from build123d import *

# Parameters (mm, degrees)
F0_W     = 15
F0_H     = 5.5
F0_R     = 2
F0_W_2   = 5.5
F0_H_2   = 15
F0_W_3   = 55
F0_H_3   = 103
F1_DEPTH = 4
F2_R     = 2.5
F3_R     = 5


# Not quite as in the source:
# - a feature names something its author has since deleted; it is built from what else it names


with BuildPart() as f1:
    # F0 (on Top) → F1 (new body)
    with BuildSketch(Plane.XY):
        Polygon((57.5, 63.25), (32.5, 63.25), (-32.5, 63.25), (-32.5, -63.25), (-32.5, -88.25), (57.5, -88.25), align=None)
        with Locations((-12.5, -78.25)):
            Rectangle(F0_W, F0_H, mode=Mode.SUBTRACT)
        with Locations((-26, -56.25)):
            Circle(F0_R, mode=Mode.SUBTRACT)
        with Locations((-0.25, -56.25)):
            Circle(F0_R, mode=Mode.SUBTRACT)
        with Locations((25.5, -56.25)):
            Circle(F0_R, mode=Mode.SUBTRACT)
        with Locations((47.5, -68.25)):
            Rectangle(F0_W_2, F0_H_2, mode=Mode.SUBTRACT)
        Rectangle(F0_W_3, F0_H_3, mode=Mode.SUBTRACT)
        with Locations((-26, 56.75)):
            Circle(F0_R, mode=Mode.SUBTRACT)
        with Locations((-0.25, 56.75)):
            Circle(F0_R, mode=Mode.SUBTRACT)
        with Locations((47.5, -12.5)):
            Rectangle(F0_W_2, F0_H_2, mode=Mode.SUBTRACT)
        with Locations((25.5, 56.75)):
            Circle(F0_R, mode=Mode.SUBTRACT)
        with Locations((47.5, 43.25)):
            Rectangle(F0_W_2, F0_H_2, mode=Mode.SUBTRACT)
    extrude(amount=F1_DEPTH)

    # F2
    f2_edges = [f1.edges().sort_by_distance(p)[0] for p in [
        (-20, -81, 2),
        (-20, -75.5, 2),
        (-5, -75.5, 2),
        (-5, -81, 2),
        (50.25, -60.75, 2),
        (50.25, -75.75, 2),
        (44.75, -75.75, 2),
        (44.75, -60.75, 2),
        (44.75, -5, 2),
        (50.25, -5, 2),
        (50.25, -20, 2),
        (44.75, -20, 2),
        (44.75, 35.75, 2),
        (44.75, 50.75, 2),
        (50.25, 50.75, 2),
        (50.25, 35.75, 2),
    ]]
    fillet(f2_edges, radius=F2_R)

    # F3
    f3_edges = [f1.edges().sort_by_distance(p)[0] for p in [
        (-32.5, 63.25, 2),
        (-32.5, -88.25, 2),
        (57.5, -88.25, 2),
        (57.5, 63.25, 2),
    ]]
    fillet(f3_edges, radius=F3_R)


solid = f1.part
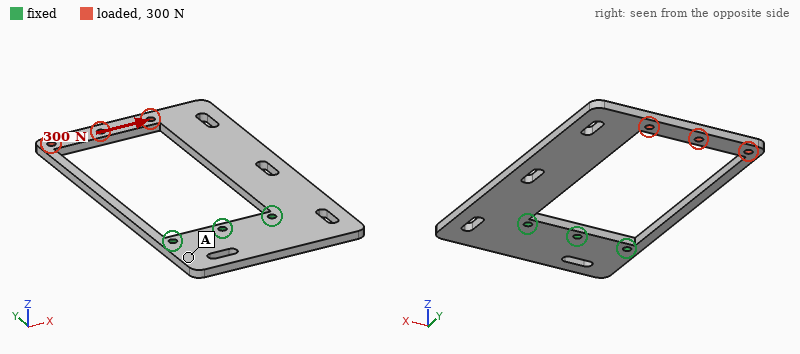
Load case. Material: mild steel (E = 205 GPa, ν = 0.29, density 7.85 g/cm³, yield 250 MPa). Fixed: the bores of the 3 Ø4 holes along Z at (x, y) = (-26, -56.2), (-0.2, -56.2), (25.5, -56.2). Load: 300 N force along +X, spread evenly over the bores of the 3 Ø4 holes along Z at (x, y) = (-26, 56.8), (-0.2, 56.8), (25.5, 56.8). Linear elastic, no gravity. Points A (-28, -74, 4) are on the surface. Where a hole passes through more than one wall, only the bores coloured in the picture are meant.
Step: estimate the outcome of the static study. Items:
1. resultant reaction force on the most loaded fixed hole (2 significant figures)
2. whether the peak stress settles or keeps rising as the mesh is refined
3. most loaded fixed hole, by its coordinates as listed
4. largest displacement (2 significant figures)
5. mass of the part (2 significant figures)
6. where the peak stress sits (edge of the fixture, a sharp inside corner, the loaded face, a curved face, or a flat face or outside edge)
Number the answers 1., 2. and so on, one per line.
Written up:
1. 1.2 kN
2. keeps rising
3. (25.5, -56.2)
4. 0.12 mm
5. 240 g
6. a sharp inside corner
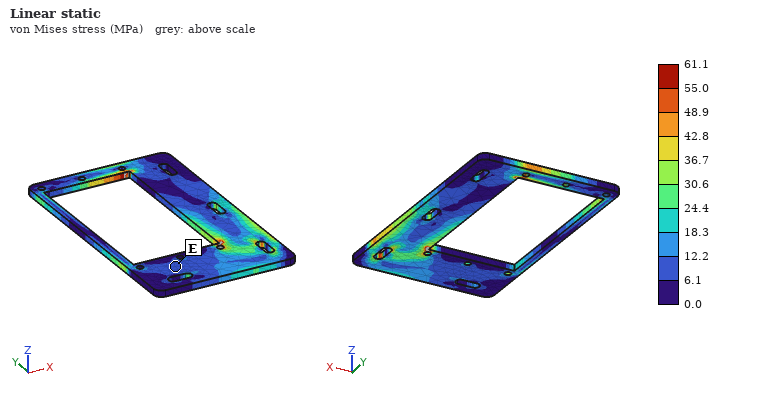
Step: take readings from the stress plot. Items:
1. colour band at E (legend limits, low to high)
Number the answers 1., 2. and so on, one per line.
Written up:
1. 6.1 to 12.2 MPa
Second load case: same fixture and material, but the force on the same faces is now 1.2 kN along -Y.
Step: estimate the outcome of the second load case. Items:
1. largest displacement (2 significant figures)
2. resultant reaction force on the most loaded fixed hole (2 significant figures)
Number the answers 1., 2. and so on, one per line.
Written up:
1. 53 µm
2. 600 N
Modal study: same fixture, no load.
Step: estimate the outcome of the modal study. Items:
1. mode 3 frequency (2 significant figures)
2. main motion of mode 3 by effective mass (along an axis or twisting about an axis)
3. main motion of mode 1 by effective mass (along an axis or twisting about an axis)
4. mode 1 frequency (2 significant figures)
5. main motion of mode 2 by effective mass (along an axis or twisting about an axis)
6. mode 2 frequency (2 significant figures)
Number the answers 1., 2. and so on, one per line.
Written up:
1. 1000 Hz
2. along X
3. along Z
4. 170 Hz
5. twisting about Y
6. 450 Hz
